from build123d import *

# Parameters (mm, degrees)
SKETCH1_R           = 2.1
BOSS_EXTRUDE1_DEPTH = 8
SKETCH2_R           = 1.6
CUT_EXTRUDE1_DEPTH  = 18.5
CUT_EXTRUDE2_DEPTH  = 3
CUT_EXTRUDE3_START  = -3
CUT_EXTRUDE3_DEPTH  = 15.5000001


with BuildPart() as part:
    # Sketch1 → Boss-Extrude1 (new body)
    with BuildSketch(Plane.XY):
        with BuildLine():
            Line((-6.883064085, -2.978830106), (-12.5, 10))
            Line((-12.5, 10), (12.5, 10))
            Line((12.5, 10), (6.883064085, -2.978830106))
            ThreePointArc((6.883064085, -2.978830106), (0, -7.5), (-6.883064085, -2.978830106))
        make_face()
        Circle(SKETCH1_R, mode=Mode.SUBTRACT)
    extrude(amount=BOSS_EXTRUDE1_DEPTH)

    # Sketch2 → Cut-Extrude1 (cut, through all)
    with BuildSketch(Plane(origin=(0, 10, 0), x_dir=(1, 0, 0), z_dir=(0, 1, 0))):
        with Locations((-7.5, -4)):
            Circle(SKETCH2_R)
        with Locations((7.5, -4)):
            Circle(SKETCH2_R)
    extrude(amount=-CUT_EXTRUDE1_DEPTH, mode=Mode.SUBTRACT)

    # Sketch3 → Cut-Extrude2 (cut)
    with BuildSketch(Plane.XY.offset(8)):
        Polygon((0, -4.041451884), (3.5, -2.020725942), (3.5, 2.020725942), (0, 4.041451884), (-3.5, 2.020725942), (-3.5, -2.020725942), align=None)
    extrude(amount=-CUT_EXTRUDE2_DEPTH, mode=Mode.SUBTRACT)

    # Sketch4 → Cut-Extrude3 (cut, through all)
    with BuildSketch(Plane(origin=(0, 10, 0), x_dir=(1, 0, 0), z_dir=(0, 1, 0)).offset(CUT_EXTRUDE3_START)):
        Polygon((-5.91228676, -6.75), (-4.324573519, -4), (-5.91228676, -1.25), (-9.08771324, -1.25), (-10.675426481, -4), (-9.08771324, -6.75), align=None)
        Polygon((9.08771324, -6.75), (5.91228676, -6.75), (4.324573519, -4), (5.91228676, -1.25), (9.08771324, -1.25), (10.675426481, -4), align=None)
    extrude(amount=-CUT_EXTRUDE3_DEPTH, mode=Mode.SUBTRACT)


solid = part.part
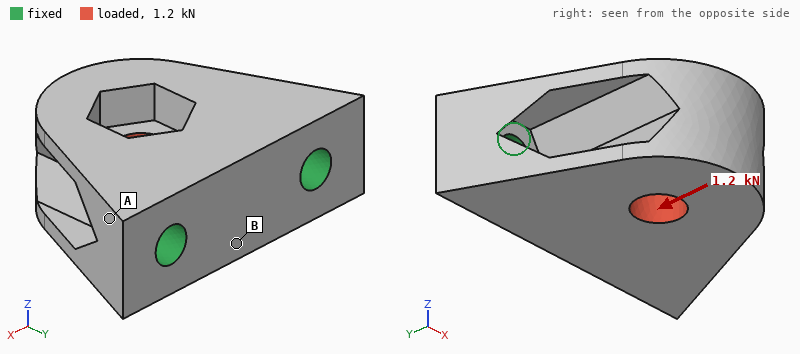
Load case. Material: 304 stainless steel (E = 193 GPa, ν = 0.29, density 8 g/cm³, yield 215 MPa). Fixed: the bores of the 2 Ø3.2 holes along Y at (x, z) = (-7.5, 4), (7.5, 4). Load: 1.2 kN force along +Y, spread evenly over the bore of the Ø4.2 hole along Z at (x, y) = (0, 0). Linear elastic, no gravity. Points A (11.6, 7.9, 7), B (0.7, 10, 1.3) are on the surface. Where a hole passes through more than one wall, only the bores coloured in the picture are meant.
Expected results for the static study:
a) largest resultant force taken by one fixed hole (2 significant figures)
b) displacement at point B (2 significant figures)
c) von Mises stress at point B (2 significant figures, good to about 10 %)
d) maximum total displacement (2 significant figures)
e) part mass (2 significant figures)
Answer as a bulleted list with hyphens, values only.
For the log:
- 630 N
- 1.8 µm
- 18 MPa
- 5.2 µm
- 14 g
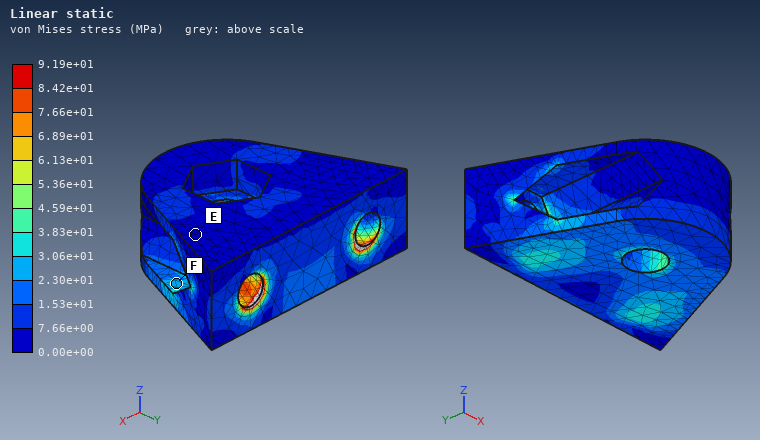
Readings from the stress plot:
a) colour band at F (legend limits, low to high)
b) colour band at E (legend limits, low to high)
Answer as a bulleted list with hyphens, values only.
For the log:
- 2.30e+01 to 3.06e+01 MPa
- 0.00e+00 to 7.66e+00 MPa
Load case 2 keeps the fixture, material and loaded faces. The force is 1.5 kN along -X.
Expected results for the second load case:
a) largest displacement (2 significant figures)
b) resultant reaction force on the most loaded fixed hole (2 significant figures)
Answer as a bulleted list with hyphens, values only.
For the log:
- 6.3 µm
- 1.1 kN
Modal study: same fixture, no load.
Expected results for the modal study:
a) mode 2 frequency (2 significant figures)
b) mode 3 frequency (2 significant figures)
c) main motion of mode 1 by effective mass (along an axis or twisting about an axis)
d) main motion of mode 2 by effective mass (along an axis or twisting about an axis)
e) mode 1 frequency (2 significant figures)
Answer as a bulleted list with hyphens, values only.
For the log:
- 30 kHz
- 36 kHz
- along Z
- along X
- 14 kHz
